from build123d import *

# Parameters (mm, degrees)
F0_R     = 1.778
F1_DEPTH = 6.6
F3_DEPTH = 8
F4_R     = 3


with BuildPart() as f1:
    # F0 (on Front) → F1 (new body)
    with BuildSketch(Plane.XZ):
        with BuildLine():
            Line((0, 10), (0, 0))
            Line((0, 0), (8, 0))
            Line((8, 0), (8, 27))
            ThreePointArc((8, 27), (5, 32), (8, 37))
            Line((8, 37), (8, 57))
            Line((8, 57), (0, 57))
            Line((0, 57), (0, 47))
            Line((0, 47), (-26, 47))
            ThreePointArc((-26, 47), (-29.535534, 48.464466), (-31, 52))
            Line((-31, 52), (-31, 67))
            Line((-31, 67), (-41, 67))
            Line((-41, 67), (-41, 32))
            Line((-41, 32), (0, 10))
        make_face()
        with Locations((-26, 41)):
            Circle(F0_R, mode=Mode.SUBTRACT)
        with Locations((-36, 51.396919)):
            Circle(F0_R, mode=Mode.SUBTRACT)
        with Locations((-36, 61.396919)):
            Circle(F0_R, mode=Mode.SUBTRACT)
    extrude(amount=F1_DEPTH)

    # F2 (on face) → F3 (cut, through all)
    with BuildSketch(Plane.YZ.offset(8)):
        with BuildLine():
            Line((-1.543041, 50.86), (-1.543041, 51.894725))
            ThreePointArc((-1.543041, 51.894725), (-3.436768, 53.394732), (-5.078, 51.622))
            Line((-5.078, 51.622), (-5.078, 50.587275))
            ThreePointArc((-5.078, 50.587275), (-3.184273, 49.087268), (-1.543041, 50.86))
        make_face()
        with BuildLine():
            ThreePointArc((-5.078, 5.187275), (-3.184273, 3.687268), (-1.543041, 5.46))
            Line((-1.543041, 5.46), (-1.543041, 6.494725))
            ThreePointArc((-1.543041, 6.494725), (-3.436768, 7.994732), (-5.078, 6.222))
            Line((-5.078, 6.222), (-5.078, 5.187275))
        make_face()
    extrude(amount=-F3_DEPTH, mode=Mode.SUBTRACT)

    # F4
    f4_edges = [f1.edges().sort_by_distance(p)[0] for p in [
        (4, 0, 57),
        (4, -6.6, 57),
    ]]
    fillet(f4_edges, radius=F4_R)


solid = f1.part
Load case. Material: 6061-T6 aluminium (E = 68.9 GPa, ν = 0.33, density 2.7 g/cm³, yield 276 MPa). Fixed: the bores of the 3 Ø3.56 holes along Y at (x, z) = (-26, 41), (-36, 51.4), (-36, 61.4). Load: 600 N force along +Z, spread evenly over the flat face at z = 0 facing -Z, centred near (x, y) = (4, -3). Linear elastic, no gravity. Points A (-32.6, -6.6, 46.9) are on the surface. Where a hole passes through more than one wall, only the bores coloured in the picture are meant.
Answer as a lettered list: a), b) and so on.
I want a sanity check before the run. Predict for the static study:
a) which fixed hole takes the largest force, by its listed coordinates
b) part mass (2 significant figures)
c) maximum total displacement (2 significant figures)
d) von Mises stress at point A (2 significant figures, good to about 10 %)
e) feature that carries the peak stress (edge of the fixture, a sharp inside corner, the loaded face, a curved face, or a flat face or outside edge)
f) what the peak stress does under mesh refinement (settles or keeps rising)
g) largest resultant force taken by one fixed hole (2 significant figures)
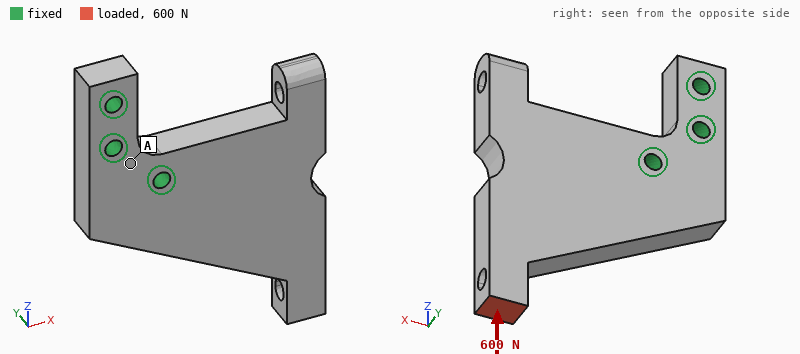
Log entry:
a) (-26, 41)
b) 29 g
c) 77 µm
d) 15 MPa
e) edge of the fixture
f) keeps rising
g) 1.6 kN
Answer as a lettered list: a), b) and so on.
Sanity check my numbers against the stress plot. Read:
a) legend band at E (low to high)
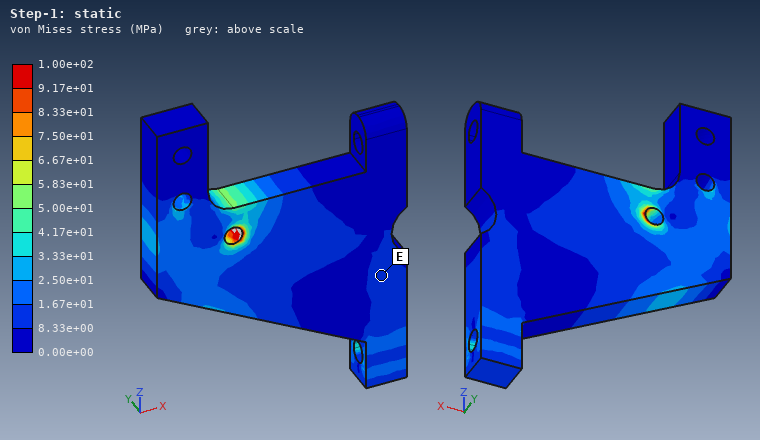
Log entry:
a) 8.33e+00 to 1.67e+01 MPa
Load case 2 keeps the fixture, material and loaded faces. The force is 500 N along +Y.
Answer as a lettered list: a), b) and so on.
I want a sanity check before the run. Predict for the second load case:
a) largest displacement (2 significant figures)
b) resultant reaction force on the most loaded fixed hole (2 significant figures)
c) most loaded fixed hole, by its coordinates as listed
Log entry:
a) 0.71 mm
b) 1.0 kN
c) (-26, 41)
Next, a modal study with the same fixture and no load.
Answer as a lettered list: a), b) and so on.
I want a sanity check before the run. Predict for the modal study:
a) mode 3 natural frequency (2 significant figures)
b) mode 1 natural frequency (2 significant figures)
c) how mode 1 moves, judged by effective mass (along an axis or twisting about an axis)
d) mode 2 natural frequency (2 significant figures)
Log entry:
a) 4900 Hz
b) 2600 Hz
c) along Y
d) 4800 Hz
